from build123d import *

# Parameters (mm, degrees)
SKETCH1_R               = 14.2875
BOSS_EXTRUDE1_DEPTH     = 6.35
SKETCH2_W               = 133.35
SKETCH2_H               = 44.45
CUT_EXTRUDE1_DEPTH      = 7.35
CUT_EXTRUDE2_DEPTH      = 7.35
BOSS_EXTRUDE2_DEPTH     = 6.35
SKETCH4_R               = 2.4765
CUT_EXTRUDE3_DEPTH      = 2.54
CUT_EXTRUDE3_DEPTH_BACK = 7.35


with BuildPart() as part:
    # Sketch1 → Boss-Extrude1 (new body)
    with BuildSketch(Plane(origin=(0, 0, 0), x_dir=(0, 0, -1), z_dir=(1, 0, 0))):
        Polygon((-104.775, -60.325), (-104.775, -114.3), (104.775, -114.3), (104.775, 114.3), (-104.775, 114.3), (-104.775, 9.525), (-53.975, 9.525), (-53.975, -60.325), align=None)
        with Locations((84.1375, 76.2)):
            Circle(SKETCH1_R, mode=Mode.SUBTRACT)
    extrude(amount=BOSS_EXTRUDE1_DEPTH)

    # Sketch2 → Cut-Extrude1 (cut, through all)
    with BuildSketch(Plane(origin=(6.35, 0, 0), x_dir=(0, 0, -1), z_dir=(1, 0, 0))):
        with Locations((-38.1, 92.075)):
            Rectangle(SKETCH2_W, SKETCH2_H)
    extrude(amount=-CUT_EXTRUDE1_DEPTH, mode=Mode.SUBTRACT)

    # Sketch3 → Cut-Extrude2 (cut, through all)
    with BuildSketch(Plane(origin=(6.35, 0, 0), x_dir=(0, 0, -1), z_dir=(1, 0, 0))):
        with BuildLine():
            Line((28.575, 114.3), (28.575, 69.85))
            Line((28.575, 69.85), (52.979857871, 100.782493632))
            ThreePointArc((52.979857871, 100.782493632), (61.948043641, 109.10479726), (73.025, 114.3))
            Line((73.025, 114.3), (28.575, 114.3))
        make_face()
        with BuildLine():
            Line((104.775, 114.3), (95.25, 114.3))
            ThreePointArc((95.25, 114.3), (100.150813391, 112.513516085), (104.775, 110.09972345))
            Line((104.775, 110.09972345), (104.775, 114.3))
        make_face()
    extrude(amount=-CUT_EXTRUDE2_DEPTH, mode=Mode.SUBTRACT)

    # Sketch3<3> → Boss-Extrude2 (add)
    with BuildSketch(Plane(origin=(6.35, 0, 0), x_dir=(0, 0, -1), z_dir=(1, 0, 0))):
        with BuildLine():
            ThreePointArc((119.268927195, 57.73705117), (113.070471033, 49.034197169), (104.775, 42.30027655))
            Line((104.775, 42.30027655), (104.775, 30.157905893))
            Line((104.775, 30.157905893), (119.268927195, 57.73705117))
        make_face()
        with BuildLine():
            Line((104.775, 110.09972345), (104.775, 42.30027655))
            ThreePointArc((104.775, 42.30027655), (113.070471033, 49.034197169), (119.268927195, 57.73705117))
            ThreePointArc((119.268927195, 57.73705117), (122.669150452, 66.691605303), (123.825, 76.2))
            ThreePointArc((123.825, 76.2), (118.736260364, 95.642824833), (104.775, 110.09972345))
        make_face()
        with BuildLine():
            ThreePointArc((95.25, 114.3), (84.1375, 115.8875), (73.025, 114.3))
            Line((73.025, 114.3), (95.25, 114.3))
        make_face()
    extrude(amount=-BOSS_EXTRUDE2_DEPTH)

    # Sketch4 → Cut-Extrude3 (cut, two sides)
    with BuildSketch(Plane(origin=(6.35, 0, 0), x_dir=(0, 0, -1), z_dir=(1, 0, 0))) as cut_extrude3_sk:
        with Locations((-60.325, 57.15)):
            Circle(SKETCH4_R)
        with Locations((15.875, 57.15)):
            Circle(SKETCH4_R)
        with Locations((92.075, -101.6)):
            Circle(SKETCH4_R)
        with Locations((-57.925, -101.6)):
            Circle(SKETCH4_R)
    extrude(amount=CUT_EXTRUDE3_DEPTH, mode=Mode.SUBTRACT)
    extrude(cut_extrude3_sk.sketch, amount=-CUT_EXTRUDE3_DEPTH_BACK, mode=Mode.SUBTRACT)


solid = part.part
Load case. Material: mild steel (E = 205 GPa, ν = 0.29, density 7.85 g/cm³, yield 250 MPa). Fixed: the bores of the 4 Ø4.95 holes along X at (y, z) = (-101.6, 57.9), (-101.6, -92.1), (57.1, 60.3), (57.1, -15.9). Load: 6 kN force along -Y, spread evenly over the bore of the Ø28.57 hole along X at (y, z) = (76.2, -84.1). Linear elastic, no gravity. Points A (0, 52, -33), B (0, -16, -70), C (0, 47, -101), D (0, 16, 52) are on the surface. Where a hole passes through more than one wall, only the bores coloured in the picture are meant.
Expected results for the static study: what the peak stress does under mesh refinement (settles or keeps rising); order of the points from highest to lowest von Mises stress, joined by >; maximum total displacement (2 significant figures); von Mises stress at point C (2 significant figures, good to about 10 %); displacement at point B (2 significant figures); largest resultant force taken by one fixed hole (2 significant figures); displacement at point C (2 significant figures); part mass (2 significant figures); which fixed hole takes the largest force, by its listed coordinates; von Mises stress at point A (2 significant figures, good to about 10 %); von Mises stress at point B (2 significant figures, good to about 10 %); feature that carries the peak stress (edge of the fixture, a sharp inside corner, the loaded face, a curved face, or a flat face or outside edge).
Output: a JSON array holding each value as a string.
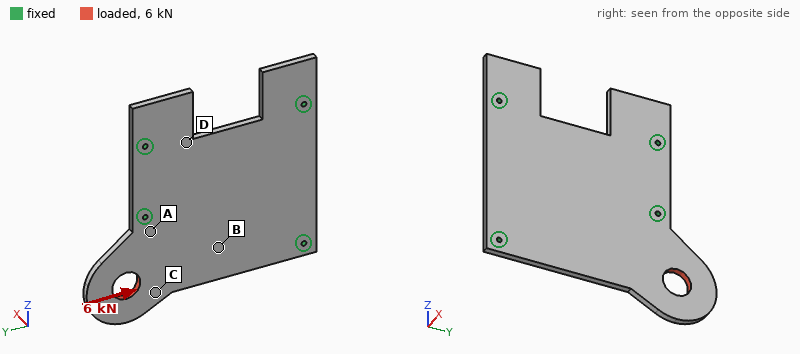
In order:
["keeps rising", "C > A > B > D", "20 µm", "21 MPa", "5.3 µm", "3.0 kN", "13 µm", "1.9 kg", "(57.1, -15.9)", "12 MPa", "9.7 MPa", "edge of the fixture"]
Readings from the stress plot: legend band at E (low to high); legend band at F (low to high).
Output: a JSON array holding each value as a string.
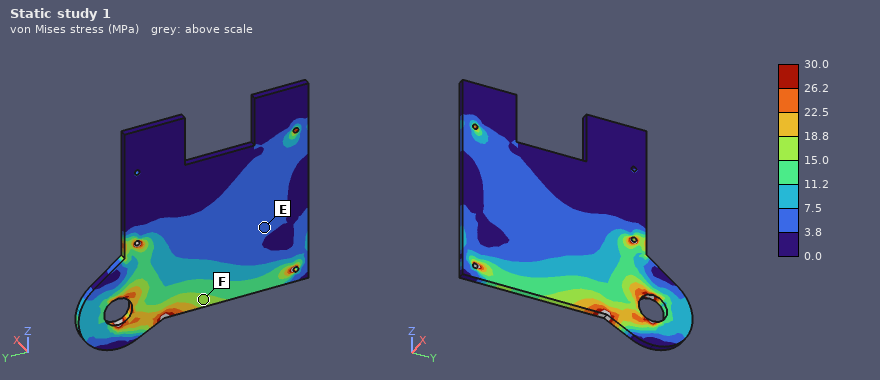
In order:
["3.8 to 7.5 MPa", "15.0 to 18.8 MPa"]
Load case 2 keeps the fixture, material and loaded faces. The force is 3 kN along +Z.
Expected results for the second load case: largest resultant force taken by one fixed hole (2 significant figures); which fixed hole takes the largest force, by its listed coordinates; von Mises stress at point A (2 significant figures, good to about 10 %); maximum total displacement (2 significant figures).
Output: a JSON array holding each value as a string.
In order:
["2.7 kN", "(57.1, -15.9)", "9.9 MPa", "11 µm"]
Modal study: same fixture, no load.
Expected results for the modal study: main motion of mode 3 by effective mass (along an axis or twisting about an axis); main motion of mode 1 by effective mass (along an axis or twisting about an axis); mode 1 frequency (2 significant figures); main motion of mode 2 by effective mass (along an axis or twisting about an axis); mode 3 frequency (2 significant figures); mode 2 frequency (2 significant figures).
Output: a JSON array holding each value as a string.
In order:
["along X", "along X", "470 Hz", "along X", "1200 Hz", "840 Hz"]
